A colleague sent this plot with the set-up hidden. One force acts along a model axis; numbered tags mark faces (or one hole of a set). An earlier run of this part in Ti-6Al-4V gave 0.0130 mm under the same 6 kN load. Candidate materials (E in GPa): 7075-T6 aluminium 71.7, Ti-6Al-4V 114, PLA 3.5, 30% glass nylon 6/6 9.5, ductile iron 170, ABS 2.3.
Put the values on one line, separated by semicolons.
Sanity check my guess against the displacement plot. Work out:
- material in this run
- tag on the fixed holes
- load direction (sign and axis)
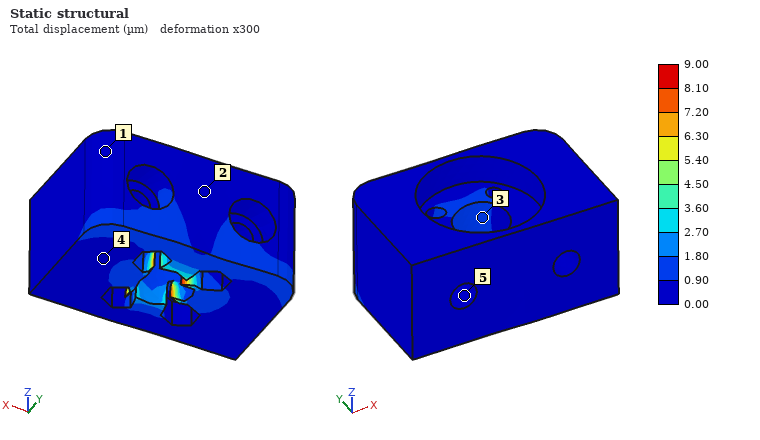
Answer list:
ductile iron; 5; +X
